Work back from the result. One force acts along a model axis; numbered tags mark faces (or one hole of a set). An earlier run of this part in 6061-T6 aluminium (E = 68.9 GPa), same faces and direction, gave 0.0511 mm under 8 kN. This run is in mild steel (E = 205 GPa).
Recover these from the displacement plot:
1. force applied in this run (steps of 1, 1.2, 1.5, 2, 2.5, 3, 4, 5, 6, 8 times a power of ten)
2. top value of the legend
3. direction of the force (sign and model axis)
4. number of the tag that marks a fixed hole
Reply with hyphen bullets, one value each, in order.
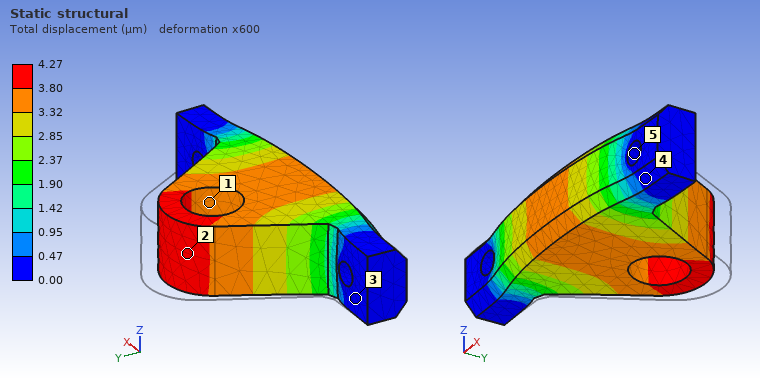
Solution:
- 2 kN
- 4.27 µm
- -Y
- 5
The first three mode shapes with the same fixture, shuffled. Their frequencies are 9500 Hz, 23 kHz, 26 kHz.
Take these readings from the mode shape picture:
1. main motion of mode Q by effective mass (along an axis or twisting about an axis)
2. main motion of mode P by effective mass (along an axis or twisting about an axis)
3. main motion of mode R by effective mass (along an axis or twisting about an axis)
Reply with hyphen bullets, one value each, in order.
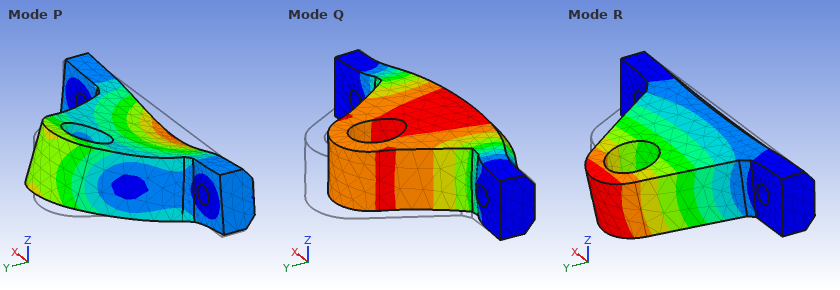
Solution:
- along Y
- along Z
- along Z
